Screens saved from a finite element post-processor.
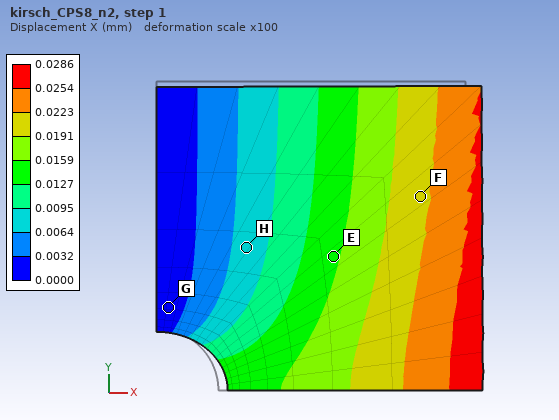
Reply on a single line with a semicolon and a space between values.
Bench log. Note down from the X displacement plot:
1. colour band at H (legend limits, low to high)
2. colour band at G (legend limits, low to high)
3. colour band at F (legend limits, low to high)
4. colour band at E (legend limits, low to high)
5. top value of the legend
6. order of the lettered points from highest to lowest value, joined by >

0.0064 to 0.0095 mm; 0.0000 to 0.0032 mm; 0.0191 to 0.0223 mm; 0.0127 to 0.0159 mm; 0.0286 mm; F > E > H > G
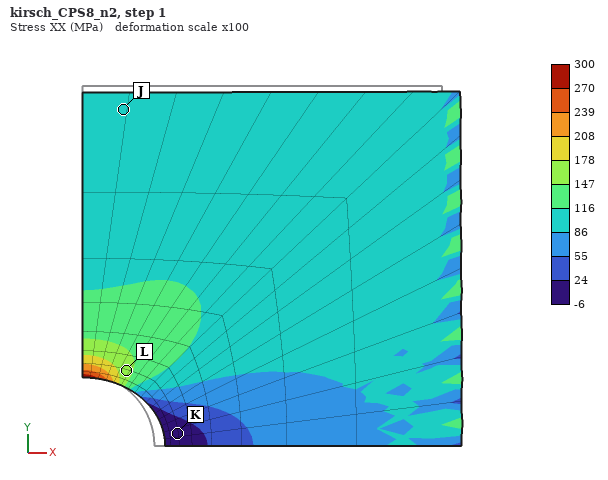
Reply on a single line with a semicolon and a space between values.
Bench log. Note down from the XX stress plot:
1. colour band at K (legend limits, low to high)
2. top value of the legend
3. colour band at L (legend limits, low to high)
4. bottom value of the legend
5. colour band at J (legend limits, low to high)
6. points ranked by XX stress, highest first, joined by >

-6 to 24 MPa; 300 MPa; 147 to 178 MPa; -6 MPa; 86 to 116 MPa; L > J > K
